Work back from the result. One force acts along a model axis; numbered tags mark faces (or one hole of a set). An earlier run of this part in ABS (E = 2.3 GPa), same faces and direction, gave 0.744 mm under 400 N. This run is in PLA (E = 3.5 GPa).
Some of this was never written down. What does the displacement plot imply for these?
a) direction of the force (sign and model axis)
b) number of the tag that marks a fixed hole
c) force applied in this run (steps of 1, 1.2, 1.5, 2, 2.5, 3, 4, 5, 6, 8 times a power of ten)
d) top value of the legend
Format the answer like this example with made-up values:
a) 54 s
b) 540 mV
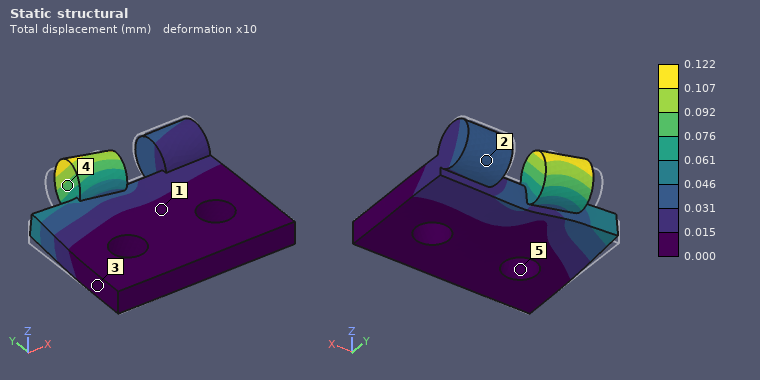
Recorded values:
a) +X
b) 5
c) 100 N
d) 0.122 mm
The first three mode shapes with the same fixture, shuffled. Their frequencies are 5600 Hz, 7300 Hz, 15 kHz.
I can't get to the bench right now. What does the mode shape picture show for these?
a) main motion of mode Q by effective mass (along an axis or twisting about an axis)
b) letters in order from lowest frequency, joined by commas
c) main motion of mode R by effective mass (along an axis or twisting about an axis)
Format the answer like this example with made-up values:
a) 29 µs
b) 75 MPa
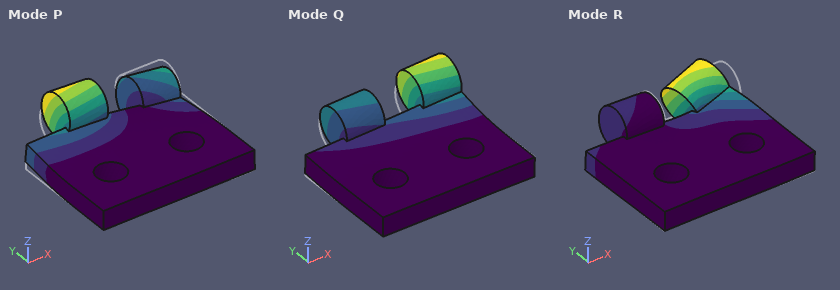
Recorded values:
a) along Z
b) Q, P, R
c) along X
